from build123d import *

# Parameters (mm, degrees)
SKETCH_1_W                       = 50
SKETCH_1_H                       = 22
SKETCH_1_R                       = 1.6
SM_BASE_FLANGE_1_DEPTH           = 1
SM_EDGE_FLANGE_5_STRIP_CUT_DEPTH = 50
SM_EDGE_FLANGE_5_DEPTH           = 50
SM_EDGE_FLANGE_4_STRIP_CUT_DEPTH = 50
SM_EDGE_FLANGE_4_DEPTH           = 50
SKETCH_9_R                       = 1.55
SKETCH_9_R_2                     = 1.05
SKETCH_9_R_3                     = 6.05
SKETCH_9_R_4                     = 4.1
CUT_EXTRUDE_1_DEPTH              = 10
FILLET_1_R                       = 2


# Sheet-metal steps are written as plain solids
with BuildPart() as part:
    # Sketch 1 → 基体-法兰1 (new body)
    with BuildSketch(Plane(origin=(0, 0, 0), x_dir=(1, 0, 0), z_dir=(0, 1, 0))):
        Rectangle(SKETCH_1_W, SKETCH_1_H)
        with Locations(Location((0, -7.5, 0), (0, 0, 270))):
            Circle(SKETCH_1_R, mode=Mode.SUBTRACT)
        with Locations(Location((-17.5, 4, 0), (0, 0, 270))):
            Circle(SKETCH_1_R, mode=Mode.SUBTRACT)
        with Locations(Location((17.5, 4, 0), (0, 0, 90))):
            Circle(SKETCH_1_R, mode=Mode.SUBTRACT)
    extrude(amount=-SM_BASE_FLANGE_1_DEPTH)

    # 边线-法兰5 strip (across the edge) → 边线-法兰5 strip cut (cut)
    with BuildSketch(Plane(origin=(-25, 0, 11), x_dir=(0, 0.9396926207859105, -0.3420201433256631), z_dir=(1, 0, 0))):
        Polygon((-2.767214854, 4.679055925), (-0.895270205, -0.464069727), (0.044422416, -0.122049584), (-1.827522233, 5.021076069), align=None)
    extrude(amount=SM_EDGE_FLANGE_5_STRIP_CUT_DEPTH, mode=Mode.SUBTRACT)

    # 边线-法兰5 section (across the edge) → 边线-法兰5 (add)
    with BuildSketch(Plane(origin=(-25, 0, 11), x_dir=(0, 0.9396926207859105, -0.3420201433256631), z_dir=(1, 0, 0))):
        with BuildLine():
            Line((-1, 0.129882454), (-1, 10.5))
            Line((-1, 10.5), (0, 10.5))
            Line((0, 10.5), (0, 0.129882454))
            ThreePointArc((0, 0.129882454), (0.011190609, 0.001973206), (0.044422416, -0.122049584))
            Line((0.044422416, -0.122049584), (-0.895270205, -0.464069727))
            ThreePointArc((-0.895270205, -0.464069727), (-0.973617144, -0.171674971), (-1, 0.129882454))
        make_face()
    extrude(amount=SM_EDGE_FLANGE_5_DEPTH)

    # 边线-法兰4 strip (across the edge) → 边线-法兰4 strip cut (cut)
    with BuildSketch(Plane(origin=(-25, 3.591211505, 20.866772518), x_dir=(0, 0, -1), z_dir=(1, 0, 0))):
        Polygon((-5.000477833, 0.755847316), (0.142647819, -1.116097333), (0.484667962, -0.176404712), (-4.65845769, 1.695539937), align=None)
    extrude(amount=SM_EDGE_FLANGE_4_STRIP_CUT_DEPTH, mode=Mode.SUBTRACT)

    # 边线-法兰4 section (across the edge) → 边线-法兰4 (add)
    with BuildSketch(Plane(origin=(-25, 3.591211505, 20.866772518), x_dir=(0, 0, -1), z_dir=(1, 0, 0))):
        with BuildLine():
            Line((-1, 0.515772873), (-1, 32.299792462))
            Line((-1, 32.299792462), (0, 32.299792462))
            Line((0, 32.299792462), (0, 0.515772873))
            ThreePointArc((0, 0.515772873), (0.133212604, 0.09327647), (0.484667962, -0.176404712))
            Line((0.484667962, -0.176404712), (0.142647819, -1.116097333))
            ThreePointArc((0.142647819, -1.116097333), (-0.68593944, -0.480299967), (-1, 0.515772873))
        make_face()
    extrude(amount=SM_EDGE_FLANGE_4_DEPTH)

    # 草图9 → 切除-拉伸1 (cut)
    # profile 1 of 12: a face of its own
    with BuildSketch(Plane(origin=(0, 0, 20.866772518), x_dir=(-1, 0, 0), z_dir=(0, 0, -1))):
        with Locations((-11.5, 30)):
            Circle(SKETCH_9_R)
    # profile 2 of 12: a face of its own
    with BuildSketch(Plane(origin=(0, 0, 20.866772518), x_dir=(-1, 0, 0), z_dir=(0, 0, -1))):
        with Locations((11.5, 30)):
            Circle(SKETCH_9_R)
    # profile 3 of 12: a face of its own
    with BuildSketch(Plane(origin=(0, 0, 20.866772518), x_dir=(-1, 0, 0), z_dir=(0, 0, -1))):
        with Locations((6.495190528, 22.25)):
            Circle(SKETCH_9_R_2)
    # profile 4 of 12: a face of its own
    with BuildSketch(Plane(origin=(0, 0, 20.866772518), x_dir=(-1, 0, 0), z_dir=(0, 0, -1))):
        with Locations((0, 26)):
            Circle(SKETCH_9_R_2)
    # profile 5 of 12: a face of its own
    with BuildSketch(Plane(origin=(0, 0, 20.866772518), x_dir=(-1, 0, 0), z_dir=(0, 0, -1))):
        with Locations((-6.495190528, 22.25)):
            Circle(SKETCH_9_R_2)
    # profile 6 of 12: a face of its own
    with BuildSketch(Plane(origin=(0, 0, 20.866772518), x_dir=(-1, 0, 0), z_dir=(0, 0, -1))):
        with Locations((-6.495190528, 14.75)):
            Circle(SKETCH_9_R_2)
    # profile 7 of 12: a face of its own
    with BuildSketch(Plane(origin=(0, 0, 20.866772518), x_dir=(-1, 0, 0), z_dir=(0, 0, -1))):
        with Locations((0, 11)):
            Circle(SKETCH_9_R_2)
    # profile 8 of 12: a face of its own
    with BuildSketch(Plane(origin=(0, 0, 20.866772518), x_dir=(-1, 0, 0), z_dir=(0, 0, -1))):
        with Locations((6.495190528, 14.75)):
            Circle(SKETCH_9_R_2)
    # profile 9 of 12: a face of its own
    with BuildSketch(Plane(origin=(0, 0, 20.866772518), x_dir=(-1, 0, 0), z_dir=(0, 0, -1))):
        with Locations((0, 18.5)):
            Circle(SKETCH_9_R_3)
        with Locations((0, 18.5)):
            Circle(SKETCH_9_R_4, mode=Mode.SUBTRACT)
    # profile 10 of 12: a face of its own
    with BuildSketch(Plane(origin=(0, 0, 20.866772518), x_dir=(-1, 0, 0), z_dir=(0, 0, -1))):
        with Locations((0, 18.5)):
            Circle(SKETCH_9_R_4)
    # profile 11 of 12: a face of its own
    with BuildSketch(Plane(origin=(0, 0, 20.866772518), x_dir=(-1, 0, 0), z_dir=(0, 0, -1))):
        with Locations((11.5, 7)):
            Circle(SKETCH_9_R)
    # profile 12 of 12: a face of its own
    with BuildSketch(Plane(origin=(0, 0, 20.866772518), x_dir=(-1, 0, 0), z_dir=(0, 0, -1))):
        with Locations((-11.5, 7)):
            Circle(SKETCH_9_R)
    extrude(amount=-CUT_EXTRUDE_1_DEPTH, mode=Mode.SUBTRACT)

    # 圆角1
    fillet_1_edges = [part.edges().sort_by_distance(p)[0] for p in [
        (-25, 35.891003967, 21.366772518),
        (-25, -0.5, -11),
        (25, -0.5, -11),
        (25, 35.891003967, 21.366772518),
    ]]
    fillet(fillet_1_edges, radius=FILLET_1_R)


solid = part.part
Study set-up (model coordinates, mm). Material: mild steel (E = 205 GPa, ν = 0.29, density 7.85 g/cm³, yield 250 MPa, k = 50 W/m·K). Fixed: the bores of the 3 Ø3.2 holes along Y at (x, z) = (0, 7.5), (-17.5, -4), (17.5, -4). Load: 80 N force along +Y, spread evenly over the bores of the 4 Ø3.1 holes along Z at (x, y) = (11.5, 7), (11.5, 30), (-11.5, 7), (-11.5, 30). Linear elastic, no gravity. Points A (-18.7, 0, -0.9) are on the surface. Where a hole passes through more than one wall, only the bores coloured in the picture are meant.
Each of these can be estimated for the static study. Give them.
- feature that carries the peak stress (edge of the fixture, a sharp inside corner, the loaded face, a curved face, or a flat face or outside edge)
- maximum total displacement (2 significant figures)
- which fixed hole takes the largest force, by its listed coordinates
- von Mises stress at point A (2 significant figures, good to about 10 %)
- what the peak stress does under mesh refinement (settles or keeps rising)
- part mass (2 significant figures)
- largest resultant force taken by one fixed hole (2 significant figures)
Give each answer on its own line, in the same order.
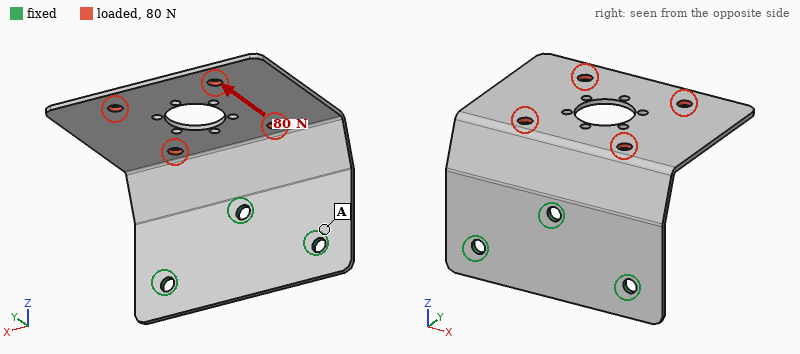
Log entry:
edge of the fixture
0.38 mm
(0, 7.5)
23 MPa
keeps rising
24 g
220 N
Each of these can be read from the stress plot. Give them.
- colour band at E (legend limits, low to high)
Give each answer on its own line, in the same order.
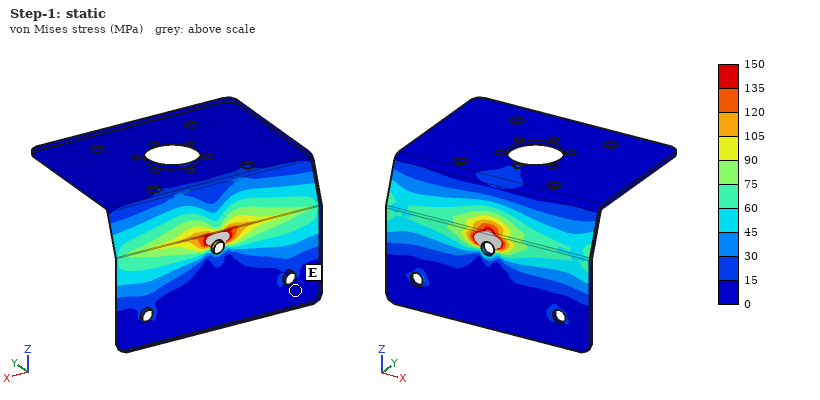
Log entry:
0 to 15 MPa
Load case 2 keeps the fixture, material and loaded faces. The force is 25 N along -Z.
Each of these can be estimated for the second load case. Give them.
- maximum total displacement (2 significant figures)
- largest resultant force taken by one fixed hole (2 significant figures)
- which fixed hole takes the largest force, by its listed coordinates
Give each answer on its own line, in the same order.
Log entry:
0.42 mm
47 N
(0, 7.5)
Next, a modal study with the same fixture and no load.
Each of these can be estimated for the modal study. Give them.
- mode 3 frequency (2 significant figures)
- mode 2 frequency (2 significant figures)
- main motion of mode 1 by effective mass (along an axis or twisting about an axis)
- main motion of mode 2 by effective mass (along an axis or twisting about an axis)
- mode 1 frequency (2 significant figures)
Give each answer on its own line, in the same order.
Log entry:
1200 Hz
650 Hz
along Z
along X
420 Hz
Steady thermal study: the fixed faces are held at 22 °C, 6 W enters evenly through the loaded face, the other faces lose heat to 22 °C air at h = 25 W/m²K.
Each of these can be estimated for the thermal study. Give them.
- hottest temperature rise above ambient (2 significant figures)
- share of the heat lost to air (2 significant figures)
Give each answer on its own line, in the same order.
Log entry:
51 K
58 %
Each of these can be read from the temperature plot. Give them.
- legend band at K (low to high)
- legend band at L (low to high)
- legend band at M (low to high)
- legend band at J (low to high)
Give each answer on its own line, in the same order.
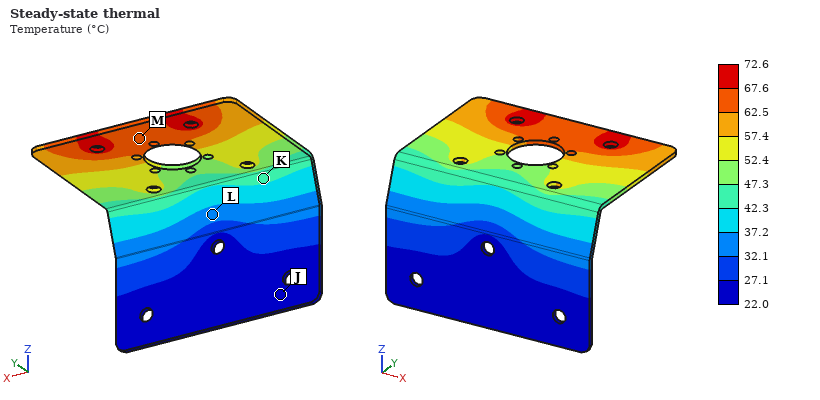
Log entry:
42.3 to 47.3 °C
32.1 to 37.2 °C
62.5 to 67.6 °C
22.0 to 27.1 °C
